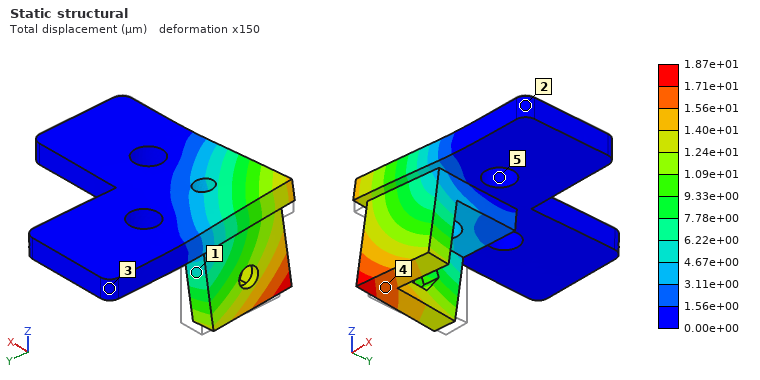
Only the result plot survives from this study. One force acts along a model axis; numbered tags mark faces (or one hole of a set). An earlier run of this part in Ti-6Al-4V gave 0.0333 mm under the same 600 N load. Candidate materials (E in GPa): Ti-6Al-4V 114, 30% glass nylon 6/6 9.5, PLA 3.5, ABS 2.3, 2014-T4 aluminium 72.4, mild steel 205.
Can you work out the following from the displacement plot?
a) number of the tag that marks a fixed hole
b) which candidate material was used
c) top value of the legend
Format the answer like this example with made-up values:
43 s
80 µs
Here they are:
5
mild steel
1.87e+01 µm
